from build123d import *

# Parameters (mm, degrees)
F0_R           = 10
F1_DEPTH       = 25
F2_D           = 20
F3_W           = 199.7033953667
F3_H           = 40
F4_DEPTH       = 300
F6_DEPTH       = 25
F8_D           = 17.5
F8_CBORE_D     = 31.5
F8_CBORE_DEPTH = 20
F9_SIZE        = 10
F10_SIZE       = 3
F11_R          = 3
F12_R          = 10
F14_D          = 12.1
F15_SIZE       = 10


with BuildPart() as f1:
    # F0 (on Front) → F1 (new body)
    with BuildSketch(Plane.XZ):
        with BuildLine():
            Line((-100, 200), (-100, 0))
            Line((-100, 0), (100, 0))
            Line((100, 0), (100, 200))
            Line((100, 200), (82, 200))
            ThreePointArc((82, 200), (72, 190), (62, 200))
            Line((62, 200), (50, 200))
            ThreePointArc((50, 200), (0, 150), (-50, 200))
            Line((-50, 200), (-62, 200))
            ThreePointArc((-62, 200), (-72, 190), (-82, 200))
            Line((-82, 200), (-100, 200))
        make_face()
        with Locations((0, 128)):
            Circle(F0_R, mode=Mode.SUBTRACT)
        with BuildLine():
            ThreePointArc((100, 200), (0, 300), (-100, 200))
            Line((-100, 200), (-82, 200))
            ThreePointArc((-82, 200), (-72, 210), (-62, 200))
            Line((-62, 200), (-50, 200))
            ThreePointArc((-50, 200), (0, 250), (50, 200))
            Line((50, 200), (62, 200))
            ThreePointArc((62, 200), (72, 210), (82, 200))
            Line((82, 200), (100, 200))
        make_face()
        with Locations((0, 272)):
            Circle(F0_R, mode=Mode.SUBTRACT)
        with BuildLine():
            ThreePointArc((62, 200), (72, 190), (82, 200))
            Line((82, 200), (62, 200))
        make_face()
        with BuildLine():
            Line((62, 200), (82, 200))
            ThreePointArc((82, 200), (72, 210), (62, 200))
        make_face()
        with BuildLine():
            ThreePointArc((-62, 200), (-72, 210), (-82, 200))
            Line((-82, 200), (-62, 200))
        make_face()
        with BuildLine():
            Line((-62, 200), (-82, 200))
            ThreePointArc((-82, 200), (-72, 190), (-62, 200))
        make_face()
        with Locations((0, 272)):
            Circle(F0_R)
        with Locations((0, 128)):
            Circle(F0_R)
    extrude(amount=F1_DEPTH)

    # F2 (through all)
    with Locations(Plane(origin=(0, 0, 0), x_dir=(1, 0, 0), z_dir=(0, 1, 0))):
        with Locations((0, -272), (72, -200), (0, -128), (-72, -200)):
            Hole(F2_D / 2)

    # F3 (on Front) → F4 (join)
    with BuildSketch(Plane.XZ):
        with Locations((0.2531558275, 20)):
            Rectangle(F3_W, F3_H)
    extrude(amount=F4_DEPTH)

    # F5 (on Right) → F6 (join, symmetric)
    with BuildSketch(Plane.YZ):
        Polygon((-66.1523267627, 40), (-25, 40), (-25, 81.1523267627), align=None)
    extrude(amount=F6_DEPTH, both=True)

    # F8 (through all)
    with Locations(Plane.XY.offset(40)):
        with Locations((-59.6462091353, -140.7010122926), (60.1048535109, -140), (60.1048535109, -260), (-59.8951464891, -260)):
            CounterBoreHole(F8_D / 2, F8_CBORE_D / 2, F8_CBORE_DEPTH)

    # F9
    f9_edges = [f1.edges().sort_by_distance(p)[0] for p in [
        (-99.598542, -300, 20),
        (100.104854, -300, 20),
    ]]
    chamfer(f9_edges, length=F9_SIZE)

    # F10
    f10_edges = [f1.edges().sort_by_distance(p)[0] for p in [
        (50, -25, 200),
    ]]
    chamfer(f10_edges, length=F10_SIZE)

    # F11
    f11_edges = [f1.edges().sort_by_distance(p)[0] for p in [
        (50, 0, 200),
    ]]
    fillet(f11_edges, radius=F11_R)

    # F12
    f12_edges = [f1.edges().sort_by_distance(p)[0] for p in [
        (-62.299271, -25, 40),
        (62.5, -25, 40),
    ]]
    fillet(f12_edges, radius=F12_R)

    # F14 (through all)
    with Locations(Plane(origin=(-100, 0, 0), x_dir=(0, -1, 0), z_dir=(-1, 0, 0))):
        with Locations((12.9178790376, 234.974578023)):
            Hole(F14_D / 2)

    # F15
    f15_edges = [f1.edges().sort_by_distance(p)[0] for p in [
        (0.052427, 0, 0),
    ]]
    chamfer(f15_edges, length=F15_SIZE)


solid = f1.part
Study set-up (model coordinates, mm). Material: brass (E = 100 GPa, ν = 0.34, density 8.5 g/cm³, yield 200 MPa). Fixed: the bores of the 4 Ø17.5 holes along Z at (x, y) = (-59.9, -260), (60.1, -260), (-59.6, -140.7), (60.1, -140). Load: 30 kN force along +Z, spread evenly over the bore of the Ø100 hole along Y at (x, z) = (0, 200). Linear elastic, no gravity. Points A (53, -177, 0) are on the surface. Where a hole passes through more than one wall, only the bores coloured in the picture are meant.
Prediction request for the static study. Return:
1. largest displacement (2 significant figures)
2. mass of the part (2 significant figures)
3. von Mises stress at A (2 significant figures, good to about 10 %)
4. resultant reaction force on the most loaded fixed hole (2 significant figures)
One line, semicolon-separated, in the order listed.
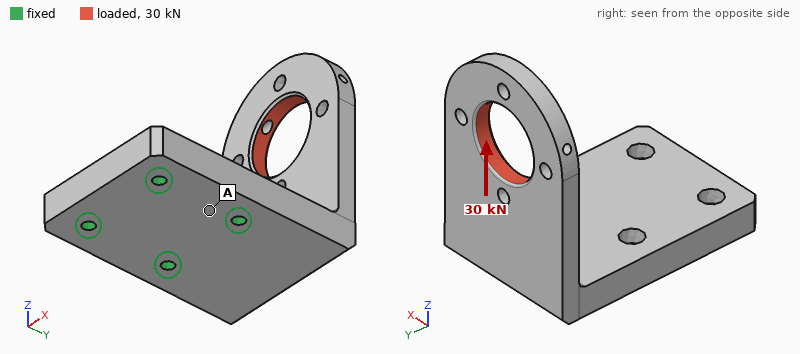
0.98 mm; 28 kg; 16 MPa; 32 kN
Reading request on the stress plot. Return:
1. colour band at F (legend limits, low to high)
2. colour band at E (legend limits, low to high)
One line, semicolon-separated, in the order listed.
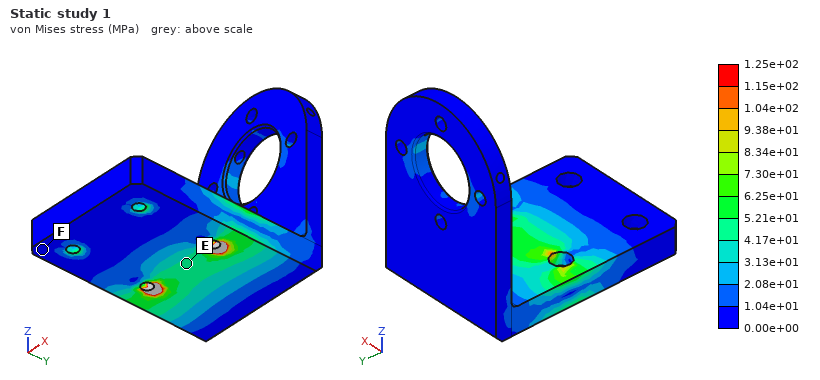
0.00e+00 to 1.04e+01 MPa; 4.17e+01 to 5.21e+01 MPa
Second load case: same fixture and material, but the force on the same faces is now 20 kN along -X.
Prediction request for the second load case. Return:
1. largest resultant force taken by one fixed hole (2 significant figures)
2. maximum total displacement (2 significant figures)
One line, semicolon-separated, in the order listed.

40 kN; 0.69 mm
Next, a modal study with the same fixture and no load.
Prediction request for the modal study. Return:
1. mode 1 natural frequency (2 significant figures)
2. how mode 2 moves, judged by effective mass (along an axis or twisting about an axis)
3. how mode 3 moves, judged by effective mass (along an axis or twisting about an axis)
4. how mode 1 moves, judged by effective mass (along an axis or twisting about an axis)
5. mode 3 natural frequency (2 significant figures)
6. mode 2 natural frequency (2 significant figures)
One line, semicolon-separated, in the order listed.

210 Hz; along X; along Z; along Y; 520 Hz; 410 Hz
